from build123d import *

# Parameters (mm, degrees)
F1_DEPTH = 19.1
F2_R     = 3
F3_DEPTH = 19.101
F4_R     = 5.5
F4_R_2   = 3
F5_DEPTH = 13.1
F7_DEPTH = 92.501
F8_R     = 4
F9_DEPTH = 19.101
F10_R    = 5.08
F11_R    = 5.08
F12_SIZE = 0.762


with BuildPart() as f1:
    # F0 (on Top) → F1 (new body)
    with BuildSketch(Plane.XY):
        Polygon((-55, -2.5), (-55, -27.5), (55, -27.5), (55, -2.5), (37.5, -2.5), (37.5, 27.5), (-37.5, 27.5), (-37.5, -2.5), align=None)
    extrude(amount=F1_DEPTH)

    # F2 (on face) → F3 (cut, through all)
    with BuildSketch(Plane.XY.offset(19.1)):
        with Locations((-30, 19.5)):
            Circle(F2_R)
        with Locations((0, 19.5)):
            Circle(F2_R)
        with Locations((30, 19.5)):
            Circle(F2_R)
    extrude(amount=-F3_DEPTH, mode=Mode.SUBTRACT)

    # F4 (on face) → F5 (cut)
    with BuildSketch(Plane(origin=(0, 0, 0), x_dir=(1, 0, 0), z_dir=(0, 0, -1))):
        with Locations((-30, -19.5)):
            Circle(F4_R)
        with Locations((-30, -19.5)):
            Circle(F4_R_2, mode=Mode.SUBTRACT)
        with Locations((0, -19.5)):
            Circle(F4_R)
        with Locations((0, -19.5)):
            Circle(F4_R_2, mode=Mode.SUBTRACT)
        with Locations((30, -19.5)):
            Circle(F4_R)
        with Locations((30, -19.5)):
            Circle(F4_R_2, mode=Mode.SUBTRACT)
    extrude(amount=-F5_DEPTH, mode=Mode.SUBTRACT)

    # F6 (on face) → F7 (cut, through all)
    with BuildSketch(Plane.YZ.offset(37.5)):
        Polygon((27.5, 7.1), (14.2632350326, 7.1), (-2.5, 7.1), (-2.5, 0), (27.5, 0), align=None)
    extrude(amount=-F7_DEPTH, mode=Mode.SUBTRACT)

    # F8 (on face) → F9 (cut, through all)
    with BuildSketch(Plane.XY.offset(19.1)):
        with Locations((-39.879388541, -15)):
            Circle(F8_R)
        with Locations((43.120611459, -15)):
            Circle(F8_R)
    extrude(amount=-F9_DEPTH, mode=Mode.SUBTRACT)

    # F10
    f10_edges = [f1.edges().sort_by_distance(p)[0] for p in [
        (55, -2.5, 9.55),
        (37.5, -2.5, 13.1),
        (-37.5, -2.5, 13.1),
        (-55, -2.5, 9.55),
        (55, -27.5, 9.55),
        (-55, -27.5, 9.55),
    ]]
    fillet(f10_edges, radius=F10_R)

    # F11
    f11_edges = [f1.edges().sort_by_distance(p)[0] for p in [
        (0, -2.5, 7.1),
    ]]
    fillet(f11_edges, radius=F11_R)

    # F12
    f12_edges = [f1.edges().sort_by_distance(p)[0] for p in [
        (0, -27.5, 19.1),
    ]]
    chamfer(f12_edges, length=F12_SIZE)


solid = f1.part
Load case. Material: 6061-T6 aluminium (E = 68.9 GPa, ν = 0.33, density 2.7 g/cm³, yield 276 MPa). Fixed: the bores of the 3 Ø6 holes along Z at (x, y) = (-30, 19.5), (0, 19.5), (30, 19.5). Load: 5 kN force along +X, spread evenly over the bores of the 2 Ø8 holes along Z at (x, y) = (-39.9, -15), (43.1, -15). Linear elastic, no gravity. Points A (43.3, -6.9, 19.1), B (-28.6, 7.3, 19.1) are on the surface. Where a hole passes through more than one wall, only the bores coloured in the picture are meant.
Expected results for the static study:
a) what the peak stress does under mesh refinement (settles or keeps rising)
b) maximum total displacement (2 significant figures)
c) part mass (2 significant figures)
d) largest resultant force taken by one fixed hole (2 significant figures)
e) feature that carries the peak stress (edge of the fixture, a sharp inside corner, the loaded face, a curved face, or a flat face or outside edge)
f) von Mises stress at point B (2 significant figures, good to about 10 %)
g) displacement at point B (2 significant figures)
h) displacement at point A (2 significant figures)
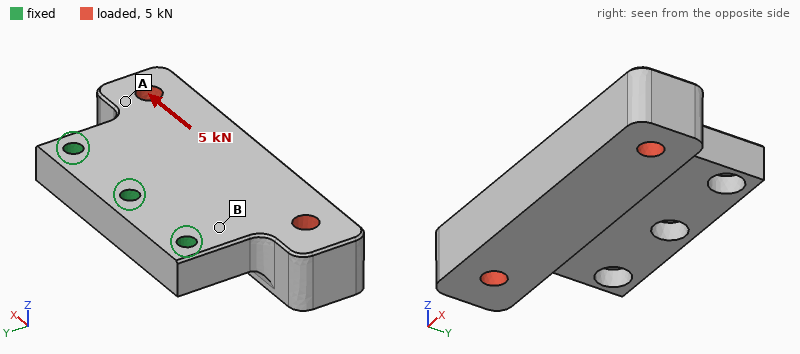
keeps rising
20 µm
200 g
3.2 kN
edge of the fixture
17 MPa
5.4 µm
14 µm
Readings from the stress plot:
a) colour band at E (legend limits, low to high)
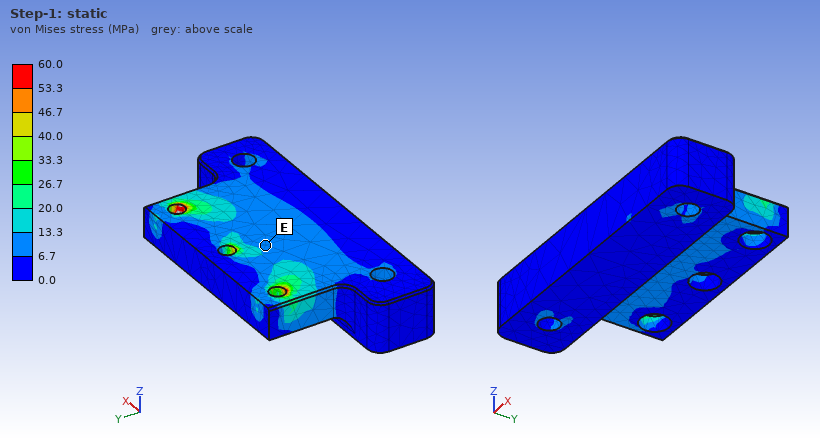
6.7 to 13.3 MPa
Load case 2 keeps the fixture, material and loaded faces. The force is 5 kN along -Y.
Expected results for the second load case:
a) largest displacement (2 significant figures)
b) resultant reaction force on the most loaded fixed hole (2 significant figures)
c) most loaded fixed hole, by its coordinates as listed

77 µm
2.0 kN
(30, 19.5)
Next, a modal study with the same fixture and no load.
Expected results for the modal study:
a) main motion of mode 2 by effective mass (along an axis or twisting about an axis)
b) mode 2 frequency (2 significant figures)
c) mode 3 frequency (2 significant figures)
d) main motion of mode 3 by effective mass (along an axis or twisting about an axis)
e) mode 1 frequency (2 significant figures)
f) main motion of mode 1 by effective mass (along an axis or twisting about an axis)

twisting about Y
3600 Hz
7400 Hz
along X
1800 Hz
along Z
